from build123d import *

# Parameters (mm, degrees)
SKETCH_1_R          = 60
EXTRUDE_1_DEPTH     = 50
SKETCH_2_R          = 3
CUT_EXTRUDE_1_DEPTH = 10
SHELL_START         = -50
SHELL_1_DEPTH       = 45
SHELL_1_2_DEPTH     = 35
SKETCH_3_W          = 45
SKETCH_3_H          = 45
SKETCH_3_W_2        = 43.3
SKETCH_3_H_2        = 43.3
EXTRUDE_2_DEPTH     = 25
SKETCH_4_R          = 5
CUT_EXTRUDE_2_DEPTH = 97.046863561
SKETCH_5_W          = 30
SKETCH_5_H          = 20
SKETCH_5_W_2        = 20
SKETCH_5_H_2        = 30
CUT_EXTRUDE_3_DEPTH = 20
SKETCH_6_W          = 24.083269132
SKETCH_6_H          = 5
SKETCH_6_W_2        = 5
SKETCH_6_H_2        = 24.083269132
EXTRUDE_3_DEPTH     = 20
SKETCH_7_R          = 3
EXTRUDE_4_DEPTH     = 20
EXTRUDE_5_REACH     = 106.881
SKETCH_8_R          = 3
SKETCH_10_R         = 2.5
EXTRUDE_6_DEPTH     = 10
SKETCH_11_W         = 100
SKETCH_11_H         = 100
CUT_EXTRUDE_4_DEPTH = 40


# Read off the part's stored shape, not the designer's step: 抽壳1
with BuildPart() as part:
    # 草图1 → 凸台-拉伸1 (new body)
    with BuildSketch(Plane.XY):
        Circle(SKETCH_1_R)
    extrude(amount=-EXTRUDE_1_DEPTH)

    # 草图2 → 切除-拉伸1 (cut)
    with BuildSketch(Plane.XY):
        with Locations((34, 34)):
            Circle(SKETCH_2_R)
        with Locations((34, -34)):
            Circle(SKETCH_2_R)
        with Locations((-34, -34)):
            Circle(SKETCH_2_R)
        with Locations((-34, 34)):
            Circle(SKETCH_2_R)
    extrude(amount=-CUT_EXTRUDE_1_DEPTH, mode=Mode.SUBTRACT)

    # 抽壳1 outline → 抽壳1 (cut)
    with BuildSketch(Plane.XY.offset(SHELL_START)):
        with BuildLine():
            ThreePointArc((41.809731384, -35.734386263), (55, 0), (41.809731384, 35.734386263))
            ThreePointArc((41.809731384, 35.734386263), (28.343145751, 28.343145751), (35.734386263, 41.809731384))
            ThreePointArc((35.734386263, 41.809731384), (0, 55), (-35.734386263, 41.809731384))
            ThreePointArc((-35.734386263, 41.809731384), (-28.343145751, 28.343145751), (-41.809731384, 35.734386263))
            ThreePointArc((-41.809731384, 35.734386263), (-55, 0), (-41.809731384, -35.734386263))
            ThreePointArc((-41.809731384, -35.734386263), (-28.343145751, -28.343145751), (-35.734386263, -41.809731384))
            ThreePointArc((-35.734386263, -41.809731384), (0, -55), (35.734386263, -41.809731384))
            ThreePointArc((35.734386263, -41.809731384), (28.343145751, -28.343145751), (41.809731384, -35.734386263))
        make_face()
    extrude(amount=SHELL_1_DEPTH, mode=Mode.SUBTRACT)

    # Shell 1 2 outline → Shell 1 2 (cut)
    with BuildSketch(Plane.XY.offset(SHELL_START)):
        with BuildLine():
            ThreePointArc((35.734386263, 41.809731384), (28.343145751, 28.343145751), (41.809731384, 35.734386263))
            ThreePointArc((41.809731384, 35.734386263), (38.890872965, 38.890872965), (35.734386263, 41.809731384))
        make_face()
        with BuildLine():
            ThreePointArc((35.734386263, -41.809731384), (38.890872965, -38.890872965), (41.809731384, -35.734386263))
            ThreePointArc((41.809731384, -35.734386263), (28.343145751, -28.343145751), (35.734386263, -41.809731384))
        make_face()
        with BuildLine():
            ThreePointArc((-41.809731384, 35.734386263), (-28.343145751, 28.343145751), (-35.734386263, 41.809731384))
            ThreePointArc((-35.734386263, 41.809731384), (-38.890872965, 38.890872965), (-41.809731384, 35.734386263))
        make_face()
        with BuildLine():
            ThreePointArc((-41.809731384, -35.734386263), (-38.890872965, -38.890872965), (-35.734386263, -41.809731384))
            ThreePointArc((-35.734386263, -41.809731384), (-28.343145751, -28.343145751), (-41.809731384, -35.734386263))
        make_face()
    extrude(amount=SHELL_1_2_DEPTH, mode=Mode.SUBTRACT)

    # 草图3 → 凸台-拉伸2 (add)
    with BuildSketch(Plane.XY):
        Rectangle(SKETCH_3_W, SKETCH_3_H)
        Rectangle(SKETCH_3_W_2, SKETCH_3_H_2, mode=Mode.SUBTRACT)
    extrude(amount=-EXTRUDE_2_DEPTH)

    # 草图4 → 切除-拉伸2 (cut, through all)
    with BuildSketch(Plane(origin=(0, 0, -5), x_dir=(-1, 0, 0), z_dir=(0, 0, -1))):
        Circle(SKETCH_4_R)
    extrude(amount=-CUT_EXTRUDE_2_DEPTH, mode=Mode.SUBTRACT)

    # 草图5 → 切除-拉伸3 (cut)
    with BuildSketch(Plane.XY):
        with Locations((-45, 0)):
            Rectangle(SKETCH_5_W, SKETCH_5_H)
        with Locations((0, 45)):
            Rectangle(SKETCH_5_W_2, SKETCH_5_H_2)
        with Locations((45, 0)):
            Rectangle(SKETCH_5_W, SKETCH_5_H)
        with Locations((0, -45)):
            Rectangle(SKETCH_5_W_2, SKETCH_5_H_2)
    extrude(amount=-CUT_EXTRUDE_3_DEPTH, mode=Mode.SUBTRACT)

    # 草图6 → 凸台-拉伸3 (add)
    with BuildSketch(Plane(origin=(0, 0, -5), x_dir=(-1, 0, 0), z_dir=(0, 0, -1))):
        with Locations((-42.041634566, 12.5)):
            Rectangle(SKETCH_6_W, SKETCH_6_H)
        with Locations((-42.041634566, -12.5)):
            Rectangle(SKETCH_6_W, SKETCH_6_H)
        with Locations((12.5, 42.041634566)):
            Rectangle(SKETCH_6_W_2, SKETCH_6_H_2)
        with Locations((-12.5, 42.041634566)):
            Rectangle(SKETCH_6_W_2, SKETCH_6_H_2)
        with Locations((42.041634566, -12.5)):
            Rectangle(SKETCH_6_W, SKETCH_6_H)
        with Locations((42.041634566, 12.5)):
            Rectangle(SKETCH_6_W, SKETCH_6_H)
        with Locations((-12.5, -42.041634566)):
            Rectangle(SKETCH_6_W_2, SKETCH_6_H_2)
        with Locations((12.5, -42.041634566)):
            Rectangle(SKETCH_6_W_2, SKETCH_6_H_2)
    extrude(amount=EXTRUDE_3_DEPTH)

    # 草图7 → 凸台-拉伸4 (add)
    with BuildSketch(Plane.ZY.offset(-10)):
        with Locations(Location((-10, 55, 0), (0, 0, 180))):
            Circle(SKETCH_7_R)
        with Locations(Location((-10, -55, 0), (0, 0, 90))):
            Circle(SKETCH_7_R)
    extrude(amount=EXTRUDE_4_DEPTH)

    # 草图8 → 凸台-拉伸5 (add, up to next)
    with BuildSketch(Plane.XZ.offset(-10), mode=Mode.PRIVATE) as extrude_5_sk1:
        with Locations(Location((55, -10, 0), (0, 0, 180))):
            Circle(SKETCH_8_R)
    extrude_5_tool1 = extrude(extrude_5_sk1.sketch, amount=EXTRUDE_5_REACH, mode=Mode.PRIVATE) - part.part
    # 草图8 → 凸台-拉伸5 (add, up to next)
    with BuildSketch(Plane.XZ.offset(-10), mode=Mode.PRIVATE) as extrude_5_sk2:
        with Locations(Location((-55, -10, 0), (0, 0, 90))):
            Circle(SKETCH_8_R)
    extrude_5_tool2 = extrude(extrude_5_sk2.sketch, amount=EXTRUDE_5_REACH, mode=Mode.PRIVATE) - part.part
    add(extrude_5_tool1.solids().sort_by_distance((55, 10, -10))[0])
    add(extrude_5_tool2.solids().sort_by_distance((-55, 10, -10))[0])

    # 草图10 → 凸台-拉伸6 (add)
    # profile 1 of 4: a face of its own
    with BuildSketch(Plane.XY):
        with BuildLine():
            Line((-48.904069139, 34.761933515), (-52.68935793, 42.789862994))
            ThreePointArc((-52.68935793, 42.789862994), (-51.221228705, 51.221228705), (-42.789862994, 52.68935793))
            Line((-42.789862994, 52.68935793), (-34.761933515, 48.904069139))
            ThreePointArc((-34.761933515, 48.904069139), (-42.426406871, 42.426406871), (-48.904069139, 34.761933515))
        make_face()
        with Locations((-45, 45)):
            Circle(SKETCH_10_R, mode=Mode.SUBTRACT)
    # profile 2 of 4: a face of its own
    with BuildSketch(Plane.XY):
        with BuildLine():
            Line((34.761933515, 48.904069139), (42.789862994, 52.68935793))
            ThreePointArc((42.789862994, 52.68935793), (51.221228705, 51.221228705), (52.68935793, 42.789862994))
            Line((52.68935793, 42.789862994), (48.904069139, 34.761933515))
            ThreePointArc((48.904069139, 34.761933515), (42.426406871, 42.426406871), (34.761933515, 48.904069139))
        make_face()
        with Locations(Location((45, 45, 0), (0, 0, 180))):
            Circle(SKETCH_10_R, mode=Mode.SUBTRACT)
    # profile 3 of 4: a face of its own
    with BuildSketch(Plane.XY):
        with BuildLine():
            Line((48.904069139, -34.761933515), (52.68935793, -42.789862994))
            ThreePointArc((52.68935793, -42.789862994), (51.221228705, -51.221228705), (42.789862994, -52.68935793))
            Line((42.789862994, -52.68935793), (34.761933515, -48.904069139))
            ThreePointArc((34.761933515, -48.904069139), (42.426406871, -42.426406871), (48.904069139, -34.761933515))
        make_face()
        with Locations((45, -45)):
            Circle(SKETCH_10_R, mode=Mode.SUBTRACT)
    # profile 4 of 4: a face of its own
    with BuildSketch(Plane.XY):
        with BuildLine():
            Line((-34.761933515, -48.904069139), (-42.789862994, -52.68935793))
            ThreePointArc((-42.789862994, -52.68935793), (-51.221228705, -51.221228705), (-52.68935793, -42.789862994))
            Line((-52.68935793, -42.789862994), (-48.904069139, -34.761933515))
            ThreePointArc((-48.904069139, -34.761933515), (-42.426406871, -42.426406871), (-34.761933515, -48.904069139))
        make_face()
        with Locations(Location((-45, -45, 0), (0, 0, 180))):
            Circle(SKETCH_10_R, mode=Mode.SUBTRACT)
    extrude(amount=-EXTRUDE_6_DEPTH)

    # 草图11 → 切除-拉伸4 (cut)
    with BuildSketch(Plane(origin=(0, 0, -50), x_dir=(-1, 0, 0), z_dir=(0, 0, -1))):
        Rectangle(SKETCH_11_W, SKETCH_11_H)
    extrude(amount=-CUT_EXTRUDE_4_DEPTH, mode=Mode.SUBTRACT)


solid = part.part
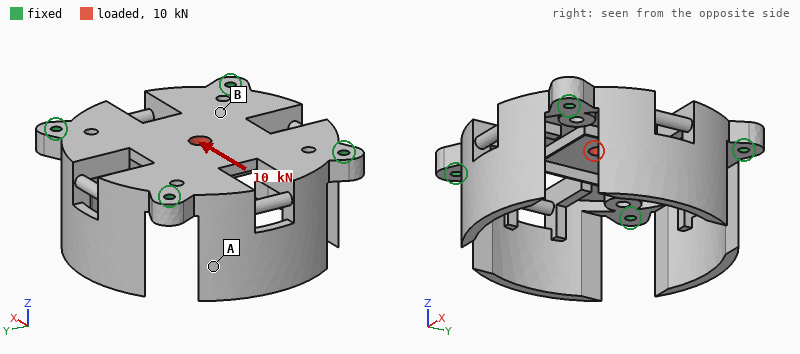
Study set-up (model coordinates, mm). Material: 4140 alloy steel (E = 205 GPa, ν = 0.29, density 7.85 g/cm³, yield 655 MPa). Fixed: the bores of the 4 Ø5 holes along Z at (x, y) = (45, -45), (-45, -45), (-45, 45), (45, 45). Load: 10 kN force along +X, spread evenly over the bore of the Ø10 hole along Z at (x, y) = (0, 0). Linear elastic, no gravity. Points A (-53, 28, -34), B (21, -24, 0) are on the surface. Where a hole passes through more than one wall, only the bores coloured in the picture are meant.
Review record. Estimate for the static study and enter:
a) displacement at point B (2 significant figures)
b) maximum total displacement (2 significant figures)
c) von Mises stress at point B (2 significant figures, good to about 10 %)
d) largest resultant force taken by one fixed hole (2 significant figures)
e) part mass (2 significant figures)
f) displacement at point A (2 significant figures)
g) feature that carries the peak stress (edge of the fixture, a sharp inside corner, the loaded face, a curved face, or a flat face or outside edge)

5.5 µm
11 µm
17 MPa
3.0 kN
890 g
3.2 µm
the loaded face
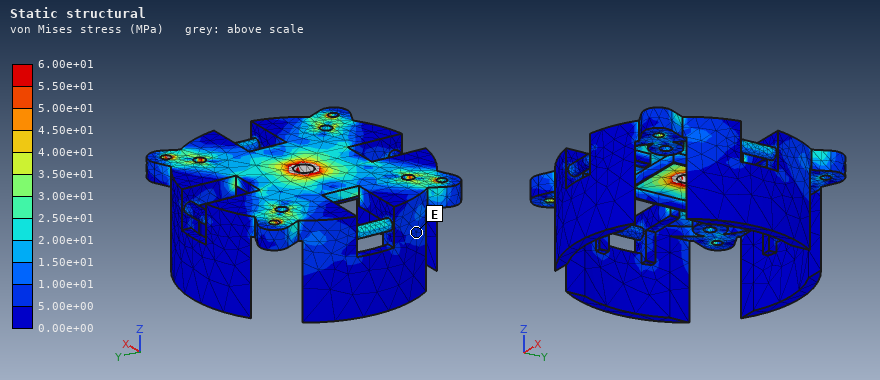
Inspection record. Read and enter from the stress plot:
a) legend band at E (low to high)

5.00e+00 to 1.00e+01 MPa
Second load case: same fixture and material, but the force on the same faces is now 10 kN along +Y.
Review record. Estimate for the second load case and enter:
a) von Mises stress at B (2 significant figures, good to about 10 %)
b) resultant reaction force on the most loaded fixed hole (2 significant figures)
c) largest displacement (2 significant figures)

16 MPa
3.0 kN
11 µm
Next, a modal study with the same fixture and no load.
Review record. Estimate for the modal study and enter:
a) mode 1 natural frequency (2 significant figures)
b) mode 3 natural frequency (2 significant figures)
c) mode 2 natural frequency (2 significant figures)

1600 Hz
1700 Hz
1700 Hz
